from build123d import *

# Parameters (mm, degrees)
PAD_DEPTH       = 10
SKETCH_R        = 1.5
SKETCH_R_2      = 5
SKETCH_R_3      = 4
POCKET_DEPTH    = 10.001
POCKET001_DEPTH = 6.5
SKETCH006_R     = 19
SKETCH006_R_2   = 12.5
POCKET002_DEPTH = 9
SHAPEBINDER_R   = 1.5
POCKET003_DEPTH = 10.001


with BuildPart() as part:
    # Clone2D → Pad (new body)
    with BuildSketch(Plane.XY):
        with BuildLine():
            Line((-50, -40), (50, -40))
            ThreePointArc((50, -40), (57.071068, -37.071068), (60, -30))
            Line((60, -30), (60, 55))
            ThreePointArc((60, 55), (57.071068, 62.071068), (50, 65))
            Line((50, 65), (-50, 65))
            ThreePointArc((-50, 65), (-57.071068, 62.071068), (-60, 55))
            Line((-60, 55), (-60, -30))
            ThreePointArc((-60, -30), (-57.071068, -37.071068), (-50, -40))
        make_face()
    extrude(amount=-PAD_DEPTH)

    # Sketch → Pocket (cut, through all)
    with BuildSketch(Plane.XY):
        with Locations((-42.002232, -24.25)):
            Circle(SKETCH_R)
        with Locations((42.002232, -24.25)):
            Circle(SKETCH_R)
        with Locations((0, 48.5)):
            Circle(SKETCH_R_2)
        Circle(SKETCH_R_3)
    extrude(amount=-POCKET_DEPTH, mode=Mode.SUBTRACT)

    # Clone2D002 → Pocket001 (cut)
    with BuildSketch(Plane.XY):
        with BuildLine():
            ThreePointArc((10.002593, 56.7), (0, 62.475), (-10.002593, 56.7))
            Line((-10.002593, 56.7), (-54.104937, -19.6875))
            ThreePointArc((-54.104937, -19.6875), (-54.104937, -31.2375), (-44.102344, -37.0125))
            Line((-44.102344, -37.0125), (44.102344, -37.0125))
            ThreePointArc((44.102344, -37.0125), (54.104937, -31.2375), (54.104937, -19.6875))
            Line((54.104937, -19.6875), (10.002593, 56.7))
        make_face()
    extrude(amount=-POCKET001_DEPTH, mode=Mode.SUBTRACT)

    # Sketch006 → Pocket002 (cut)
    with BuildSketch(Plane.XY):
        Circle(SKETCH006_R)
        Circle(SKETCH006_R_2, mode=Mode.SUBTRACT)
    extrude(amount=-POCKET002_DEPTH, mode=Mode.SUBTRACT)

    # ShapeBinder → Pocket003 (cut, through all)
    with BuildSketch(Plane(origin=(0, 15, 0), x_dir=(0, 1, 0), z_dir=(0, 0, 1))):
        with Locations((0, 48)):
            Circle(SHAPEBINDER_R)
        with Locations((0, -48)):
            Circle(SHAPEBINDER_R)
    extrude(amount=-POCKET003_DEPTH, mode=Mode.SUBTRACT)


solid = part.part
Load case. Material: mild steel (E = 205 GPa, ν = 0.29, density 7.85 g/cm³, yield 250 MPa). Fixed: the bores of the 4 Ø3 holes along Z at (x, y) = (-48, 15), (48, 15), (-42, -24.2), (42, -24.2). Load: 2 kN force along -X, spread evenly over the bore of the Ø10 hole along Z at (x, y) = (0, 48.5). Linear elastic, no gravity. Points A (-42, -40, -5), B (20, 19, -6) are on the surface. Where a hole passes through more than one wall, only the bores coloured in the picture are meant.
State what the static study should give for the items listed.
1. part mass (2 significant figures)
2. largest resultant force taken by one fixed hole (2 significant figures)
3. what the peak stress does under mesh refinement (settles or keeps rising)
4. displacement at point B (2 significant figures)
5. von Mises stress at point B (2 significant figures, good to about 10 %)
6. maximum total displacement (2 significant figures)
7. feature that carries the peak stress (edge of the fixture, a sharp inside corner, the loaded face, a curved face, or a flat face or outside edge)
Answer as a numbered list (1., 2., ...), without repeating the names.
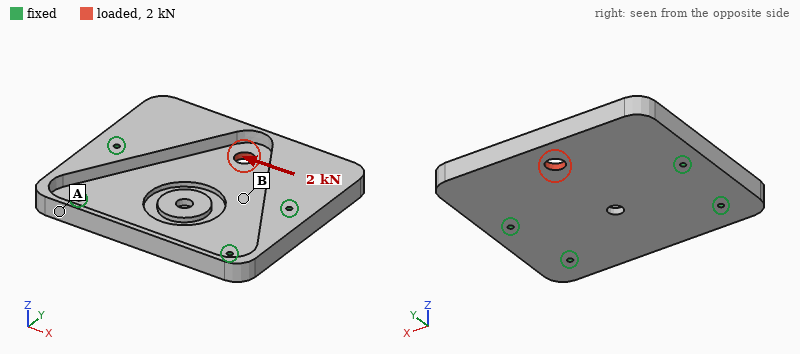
1. 620 g
2. 1.2 kN
3. keeps rising
4. 0.92 µm
5. 6.4 MPa
6. 3.5 µm
7. edge of the fixture
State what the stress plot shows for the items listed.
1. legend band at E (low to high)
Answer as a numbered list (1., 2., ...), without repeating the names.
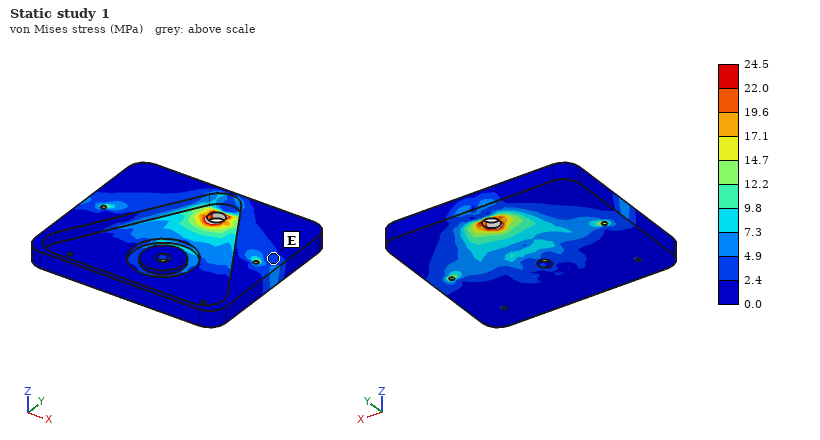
1. 2.4 to 4.9 MPa
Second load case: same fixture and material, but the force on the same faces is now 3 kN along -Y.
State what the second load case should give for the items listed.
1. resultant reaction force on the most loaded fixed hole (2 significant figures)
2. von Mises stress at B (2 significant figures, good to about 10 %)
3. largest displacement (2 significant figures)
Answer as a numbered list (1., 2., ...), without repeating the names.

1. 1.2 kN
2. 9.7 MPa
3. 11 µm
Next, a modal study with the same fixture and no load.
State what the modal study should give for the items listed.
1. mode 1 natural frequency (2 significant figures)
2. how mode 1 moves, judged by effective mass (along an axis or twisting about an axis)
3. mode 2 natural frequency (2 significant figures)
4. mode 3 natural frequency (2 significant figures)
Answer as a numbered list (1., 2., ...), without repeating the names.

1. 2000 Hz
2. along Z
3. 3300 Hz
4. 3300 Hz
